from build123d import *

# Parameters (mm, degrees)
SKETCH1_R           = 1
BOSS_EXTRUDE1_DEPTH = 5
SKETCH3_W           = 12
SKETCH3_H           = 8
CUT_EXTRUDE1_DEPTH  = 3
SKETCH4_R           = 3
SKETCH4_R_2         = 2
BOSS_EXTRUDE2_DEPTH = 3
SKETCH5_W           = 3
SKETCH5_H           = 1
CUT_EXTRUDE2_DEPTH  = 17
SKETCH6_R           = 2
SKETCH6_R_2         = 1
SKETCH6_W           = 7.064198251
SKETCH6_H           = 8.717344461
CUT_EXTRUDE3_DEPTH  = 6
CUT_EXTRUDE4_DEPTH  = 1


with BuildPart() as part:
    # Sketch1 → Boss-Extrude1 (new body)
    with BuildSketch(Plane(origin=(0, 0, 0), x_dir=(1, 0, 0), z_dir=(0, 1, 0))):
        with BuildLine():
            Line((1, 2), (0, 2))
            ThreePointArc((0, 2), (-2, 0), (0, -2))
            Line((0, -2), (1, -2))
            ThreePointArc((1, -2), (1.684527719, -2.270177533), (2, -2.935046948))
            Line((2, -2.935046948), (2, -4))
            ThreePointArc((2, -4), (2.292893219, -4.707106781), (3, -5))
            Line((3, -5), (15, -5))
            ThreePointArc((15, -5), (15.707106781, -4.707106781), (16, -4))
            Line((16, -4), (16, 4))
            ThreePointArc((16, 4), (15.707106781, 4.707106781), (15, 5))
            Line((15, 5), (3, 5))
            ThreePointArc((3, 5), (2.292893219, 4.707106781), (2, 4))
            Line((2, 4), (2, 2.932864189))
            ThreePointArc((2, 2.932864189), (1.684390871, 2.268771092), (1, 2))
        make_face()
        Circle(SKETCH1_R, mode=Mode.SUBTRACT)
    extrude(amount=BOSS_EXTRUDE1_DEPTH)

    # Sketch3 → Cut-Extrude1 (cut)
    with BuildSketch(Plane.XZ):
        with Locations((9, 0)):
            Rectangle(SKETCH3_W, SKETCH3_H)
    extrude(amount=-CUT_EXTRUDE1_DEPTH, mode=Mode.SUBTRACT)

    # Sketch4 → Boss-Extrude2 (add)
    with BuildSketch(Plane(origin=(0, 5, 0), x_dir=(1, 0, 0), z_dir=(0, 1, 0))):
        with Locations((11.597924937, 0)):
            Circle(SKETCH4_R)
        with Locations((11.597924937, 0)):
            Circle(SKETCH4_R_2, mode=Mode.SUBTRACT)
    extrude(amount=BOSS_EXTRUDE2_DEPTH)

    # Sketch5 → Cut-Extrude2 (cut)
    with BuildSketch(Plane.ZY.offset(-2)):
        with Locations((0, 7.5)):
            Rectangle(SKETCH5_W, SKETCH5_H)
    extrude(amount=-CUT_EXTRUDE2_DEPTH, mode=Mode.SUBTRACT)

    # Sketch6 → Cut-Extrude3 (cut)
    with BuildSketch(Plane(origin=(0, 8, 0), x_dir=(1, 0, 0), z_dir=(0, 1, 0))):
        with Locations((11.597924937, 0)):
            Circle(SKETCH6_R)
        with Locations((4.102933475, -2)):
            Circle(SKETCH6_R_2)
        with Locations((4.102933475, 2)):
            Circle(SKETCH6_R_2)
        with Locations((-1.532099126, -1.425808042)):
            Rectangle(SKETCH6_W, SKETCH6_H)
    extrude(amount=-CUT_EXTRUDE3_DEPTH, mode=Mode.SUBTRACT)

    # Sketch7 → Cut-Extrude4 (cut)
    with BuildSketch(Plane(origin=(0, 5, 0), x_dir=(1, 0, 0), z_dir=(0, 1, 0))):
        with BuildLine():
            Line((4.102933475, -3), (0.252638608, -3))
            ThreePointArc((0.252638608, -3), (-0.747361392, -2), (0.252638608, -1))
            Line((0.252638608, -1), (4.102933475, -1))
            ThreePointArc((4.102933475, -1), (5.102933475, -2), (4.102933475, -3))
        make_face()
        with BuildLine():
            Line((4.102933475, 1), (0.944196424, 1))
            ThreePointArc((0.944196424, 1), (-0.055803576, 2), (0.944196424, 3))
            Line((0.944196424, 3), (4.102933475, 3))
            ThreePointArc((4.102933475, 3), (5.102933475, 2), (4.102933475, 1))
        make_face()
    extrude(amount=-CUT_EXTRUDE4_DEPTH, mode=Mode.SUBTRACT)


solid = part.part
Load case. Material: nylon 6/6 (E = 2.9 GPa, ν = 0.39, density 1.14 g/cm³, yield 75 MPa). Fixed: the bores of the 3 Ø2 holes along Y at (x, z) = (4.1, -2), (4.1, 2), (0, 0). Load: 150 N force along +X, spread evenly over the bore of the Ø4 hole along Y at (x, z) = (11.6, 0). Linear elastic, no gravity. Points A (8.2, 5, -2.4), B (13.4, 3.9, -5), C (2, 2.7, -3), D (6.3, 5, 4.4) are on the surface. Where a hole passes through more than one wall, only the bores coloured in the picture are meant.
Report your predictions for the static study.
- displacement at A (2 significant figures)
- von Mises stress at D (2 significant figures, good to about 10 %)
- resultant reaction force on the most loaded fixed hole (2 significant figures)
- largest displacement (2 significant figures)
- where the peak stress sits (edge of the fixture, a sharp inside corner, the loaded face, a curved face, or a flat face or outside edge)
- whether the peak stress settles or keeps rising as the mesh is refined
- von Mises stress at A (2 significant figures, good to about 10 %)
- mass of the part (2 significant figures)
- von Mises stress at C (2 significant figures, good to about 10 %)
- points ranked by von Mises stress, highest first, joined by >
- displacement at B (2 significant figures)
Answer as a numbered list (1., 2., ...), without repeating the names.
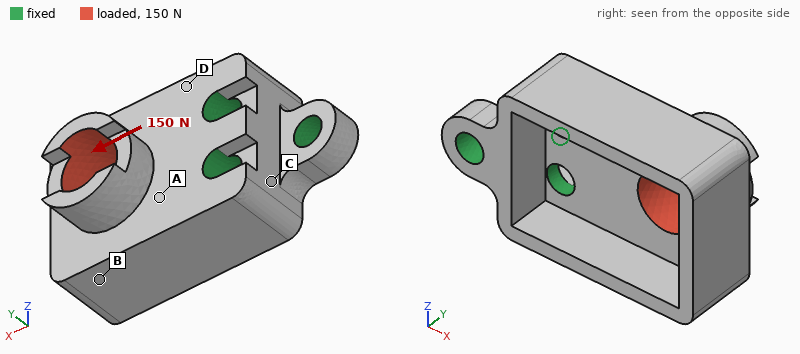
1. 0.046 mm
2. 15 MPa
3. 80 N
4. 0.23 mm
5. edge of the fixture
6. keeps rising
7. 21 MPa
8. 0.49 g
9. 9.1 MPa
10. A > D > C > B
11. 0.15 mm
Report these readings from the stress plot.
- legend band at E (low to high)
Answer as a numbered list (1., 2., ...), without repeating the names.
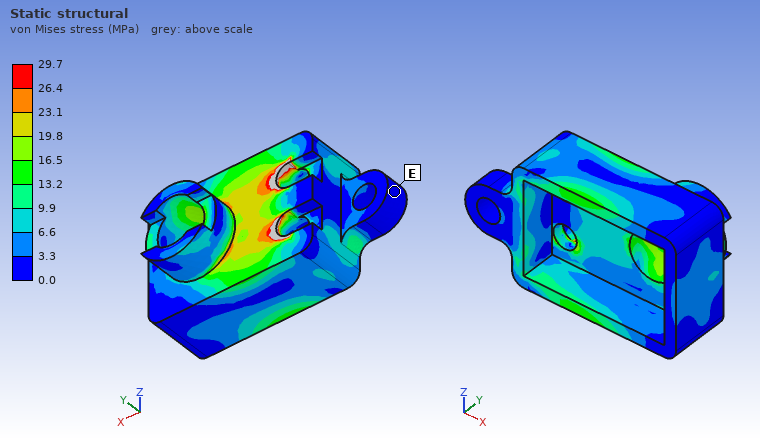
1. 0.0 to 3.3 MPa
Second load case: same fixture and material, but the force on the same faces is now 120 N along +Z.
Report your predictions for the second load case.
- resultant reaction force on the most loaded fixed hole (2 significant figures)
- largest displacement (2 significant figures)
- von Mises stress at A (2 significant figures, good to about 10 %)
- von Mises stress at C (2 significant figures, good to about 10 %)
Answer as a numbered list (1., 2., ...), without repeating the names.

1. 150 N
2. 0.21 mm
3. 16 MPa
4. 12 MPa
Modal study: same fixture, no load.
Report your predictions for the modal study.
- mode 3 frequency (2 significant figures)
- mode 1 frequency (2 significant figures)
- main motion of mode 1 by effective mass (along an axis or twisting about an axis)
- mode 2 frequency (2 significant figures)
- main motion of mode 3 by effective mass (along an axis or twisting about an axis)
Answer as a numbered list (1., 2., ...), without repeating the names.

1. 8800 Hz
2. 4300 Hz
3. along Y
4. 6400 Hz
5. along Z
